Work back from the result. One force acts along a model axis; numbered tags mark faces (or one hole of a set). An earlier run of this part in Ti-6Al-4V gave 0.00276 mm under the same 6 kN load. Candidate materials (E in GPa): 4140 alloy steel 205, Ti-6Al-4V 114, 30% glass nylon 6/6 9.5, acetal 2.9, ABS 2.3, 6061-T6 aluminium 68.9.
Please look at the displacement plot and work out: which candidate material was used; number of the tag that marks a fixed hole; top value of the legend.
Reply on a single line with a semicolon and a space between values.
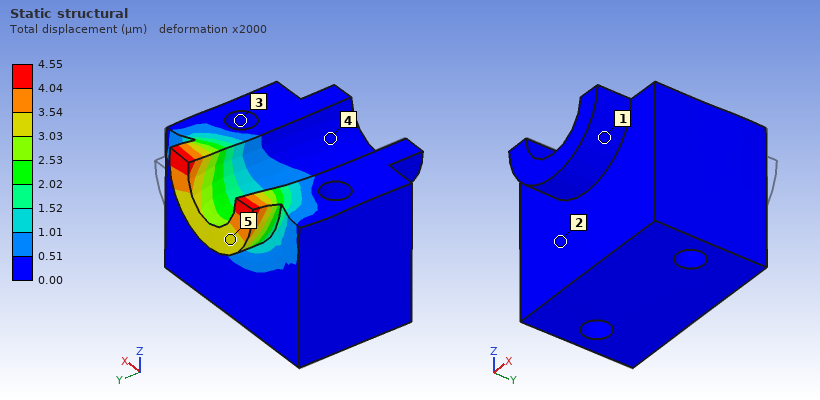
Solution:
6061-T6 aluminium; 3; 4.55 µm
